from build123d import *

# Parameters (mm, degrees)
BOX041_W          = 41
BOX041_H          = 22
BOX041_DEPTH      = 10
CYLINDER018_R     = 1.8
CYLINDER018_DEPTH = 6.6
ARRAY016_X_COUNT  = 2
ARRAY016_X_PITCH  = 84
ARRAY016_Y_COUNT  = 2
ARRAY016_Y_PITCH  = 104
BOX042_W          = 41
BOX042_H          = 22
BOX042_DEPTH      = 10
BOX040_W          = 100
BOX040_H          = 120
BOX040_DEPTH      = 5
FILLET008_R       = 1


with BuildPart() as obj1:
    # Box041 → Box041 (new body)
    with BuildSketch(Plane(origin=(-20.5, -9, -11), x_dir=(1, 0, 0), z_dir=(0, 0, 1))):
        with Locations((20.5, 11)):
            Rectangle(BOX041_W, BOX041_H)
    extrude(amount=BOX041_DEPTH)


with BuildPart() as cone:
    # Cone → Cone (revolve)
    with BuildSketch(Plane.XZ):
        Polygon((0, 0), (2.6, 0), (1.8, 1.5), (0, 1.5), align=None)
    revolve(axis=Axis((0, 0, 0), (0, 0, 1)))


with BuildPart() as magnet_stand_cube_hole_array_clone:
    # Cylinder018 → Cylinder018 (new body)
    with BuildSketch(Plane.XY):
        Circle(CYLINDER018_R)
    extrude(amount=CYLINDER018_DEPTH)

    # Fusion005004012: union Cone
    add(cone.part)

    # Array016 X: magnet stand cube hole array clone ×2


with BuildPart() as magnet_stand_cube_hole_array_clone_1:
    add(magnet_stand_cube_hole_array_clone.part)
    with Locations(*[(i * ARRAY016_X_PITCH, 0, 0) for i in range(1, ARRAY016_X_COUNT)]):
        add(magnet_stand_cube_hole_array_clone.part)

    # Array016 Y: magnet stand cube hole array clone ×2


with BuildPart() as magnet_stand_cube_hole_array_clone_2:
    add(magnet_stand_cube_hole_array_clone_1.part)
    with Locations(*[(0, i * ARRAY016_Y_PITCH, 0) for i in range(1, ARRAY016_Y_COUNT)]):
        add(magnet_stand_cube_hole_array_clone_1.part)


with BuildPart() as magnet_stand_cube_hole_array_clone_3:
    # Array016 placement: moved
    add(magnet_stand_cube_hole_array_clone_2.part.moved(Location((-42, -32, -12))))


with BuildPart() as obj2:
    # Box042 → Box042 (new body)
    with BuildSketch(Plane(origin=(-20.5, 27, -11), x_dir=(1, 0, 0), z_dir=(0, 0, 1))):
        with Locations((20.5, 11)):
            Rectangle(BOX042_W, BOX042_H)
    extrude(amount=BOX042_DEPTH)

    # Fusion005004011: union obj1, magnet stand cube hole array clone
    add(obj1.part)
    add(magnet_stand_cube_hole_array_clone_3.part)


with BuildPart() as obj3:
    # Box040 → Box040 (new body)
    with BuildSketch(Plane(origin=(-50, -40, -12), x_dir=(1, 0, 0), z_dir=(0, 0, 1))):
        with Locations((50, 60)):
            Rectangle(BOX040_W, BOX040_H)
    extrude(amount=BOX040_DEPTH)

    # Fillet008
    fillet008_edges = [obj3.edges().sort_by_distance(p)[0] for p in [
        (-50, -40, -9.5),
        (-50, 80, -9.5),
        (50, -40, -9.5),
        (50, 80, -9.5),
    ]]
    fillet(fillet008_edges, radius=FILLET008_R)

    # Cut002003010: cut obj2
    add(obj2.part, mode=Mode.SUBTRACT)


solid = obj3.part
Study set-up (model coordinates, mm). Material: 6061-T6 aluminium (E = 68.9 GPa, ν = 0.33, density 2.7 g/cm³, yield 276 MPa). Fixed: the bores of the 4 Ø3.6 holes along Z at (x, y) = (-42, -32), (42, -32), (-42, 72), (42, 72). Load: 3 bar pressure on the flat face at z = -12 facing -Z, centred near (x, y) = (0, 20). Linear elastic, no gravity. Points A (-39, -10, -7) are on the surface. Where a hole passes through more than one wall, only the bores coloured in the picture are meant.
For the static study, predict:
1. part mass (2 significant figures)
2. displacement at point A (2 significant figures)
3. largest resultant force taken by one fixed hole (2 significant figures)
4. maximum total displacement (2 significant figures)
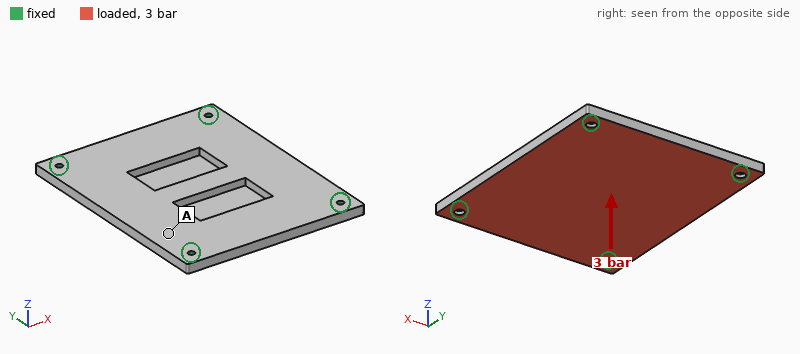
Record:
140 g
0.14 mm
1.3 kN
0.40 mm
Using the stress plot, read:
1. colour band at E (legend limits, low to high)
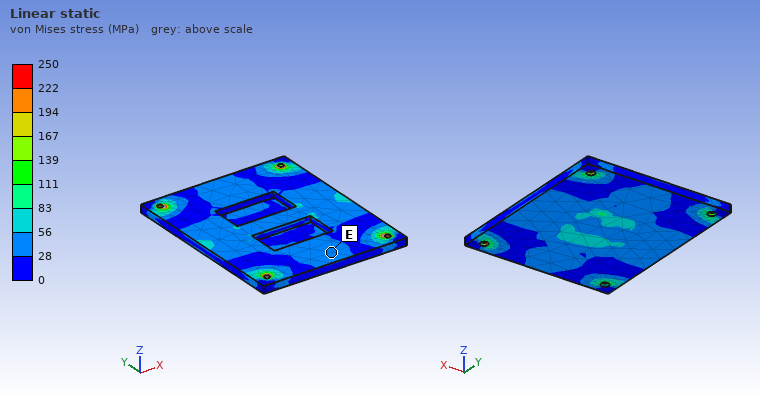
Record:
28 to 56 MPa
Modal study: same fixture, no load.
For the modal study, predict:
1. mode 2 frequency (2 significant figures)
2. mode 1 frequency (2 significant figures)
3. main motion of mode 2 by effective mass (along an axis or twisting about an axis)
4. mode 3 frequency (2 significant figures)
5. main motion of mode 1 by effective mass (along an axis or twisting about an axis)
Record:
2500 Hz
1700 Hz
twisting about Y
3200 Hz
along Z
